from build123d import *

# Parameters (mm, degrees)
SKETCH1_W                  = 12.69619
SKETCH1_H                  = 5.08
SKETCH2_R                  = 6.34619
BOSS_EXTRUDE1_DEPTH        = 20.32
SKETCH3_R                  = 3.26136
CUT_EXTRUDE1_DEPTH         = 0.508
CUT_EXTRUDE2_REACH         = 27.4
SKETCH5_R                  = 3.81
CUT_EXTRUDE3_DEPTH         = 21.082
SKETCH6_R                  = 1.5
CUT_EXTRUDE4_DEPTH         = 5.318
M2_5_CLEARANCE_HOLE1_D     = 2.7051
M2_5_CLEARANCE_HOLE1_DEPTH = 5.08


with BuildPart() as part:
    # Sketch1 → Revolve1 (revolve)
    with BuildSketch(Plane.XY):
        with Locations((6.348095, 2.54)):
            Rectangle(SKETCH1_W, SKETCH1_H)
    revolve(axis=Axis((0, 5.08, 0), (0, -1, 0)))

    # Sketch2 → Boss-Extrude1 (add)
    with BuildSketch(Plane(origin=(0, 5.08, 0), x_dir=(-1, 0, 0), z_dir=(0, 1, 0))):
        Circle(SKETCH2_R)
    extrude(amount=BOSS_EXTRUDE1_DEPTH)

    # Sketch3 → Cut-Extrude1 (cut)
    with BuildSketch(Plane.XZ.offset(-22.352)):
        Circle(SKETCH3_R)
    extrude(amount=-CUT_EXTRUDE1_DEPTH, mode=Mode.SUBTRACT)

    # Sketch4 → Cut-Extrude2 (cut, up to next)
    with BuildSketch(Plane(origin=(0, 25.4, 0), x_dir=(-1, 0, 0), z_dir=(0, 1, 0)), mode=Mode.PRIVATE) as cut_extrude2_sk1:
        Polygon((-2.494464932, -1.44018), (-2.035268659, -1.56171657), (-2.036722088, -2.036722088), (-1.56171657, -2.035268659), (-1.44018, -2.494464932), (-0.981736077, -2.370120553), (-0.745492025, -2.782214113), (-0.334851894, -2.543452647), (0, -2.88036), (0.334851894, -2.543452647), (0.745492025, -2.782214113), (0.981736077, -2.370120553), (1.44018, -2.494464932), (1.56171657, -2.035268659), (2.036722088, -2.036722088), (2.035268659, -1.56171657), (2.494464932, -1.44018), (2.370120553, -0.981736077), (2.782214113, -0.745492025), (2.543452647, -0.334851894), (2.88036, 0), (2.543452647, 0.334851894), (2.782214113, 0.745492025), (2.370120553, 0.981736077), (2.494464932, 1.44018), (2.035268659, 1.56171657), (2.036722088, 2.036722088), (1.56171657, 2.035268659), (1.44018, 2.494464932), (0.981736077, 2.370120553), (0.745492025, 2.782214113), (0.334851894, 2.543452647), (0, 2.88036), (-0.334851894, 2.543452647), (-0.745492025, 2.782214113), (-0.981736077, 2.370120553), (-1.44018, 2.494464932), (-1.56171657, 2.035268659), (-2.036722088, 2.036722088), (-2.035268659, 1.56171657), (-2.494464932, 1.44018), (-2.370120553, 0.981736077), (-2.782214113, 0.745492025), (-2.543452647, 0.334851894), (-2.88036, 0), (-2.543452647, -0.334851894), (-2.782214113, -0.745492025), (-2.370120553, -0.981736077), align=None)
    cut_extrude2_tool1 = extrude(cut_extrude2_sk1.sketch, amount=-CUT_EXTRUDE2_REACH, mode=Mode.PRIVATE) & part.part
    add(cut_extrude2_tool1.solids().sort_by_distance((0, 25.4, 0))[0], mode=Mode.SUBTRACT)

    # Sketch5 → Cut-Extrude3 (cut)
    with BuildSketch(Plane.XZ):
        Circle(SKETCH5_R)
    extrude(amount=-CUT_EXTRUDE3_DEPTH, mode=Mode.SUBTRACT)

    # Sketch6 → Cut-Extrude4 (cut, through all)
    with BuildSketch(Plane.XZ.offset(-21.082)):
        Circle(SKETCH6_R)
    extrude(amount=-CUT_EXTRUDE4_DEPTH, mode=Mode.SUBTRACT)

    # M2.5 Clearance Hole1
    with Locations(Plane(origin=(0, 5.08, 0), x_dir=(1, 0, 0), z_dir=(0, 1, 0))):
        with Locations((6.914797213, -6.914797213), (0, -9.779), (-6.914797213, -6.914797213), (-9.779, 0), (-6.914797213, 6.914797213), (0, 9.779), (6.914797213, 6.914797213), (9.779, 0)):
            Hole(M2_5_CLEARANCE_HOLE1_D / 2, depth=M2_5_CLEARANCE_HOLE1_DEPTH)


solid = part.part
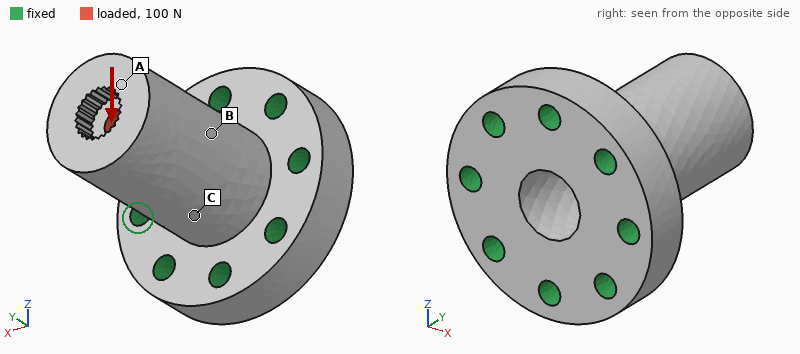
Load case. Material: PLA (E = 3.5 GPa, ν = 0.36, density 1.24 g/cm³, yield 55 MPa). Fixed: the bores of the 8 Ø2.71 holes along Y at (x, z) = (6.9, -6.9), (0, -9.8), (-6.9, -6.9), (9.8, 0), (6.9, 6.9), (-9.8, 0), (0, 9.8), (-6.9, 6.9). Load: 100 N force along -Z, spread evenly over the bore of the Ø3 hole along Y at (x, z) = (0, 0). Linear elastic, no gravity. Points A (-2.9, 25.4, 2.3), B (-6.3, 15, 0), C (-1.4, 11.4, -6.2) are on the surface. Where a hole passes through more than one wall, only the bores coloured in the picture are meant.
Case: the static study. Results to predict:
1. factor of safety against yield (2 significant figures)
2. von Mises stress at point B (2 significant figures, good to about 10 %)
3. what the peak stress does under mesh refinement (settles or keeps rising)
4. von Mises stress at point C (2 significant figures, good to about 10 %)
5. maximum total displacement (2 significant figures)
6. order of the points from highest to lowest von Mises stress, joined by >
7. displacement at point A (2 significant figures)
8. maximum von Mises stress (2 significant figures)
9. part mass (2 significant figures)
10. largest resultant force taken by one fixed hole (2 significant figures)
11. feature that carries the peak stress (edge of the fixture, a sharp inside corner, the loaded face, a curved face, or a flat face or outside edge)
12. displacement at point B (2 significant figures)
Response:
3.8
3.4 MPa
settles
5.5 MPa
0.11 mm
C > B > A
0.11 mm
15 MPa
4.8 g
66 N
the loaded face
0.047 mm
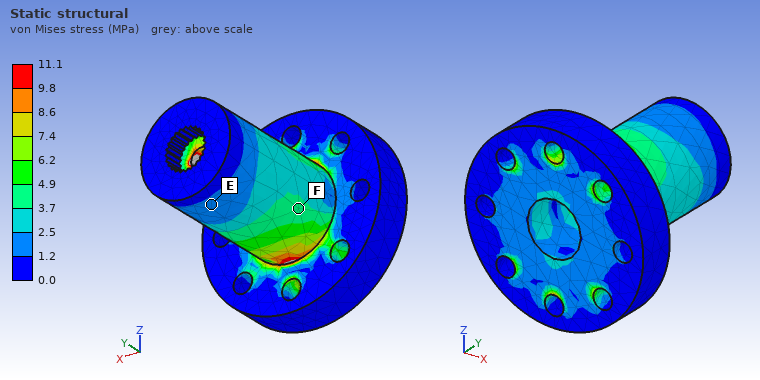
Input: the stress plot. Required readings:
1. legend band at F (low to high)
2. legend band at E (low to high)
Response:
3.7 to 4.9 MPa
1.2 to 2.5 MPa
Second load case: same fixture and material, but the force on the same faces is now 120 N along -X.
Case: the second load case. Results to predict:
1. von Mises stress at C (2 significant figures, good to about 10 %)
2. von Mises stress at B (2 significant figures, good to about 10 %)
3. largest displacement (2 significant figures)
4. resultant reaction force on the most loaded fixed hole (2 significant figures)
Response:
4.1 MPa
4.7 MPa
0.14 mm
79 N
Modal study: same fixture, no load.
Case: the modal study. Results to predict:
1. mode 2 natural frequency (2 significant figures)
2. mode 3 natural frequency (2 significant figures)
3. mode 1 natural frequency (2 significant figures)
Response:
4900 Hz
11 kHz
4900 Hz
